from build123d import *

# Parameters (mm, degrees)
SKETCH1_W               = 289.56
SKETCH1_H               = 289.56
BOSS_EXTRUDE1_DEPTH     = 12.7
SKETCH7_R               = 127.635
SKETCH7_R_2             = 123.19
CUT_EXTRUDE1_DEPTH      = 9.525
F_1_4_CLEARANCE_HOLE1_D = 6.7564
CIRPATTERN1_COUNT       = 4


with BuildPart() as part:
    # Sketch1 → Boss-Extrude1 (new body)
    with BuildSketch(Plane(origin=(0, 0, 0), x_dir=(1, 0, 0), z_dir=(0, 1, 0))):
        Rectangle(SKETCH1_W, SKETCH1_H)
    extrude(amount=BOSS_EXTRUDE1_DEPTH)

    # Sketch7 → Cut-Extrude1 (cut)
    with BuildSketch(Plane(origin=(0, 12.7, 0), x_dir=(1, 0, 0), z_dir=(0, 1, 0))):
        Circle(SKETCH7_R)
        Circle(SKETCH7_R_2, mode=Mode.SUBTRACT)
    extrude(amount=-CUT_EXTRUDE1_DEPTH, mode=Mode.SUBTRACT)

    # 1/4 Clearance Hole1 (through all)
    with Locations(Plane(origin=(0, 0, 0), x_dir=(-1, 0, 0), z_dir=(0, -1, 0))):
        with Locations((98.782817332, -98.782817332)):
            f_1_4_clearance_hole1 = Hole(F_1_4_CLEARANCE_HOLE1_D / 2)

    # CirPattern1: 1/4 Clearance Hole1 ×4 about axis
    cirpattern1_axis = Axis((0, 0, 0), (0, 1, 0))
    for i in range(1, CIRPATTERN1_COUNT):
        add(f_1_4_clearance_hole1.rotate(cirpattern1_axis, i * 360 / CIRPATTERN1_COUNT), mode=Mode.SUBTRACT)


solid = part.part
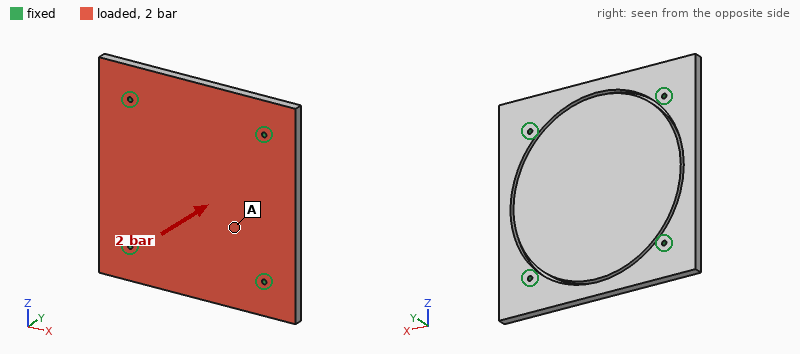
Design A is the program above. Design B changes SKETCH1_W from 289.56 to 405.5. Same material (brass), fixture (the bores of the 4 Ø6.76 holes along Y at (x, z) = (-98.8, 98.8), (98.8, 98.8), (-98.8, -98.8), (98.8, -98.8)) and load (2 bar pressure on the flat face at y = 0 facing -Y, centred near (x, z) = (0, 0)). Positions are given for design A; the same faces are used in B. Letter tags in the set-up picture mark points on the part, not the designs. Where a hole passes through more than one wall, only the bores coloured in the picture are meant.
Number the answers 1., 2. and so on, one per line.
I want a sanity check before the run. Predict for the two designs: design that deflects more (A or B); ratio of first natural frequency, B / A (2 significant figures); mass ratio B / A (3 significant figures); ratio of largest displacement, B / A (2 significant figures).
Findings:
1. B
2. 0.66
3. 1.41
4. 2.3
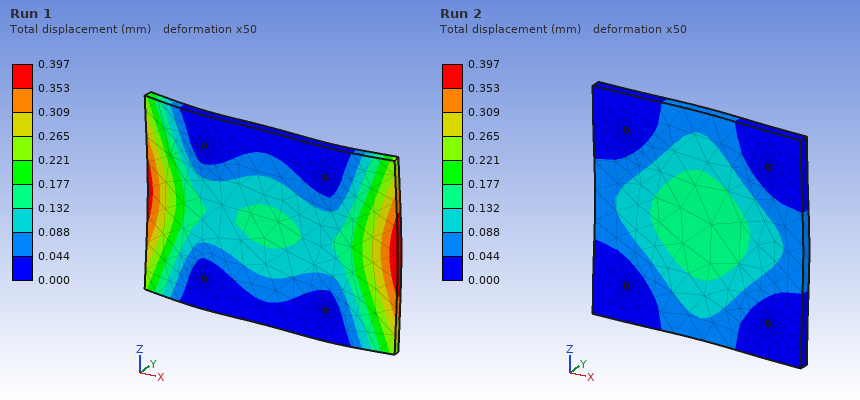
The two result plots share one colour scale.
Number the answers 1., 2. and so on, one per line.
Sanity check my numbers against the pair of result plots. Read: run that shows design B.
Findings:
1. Run 1
